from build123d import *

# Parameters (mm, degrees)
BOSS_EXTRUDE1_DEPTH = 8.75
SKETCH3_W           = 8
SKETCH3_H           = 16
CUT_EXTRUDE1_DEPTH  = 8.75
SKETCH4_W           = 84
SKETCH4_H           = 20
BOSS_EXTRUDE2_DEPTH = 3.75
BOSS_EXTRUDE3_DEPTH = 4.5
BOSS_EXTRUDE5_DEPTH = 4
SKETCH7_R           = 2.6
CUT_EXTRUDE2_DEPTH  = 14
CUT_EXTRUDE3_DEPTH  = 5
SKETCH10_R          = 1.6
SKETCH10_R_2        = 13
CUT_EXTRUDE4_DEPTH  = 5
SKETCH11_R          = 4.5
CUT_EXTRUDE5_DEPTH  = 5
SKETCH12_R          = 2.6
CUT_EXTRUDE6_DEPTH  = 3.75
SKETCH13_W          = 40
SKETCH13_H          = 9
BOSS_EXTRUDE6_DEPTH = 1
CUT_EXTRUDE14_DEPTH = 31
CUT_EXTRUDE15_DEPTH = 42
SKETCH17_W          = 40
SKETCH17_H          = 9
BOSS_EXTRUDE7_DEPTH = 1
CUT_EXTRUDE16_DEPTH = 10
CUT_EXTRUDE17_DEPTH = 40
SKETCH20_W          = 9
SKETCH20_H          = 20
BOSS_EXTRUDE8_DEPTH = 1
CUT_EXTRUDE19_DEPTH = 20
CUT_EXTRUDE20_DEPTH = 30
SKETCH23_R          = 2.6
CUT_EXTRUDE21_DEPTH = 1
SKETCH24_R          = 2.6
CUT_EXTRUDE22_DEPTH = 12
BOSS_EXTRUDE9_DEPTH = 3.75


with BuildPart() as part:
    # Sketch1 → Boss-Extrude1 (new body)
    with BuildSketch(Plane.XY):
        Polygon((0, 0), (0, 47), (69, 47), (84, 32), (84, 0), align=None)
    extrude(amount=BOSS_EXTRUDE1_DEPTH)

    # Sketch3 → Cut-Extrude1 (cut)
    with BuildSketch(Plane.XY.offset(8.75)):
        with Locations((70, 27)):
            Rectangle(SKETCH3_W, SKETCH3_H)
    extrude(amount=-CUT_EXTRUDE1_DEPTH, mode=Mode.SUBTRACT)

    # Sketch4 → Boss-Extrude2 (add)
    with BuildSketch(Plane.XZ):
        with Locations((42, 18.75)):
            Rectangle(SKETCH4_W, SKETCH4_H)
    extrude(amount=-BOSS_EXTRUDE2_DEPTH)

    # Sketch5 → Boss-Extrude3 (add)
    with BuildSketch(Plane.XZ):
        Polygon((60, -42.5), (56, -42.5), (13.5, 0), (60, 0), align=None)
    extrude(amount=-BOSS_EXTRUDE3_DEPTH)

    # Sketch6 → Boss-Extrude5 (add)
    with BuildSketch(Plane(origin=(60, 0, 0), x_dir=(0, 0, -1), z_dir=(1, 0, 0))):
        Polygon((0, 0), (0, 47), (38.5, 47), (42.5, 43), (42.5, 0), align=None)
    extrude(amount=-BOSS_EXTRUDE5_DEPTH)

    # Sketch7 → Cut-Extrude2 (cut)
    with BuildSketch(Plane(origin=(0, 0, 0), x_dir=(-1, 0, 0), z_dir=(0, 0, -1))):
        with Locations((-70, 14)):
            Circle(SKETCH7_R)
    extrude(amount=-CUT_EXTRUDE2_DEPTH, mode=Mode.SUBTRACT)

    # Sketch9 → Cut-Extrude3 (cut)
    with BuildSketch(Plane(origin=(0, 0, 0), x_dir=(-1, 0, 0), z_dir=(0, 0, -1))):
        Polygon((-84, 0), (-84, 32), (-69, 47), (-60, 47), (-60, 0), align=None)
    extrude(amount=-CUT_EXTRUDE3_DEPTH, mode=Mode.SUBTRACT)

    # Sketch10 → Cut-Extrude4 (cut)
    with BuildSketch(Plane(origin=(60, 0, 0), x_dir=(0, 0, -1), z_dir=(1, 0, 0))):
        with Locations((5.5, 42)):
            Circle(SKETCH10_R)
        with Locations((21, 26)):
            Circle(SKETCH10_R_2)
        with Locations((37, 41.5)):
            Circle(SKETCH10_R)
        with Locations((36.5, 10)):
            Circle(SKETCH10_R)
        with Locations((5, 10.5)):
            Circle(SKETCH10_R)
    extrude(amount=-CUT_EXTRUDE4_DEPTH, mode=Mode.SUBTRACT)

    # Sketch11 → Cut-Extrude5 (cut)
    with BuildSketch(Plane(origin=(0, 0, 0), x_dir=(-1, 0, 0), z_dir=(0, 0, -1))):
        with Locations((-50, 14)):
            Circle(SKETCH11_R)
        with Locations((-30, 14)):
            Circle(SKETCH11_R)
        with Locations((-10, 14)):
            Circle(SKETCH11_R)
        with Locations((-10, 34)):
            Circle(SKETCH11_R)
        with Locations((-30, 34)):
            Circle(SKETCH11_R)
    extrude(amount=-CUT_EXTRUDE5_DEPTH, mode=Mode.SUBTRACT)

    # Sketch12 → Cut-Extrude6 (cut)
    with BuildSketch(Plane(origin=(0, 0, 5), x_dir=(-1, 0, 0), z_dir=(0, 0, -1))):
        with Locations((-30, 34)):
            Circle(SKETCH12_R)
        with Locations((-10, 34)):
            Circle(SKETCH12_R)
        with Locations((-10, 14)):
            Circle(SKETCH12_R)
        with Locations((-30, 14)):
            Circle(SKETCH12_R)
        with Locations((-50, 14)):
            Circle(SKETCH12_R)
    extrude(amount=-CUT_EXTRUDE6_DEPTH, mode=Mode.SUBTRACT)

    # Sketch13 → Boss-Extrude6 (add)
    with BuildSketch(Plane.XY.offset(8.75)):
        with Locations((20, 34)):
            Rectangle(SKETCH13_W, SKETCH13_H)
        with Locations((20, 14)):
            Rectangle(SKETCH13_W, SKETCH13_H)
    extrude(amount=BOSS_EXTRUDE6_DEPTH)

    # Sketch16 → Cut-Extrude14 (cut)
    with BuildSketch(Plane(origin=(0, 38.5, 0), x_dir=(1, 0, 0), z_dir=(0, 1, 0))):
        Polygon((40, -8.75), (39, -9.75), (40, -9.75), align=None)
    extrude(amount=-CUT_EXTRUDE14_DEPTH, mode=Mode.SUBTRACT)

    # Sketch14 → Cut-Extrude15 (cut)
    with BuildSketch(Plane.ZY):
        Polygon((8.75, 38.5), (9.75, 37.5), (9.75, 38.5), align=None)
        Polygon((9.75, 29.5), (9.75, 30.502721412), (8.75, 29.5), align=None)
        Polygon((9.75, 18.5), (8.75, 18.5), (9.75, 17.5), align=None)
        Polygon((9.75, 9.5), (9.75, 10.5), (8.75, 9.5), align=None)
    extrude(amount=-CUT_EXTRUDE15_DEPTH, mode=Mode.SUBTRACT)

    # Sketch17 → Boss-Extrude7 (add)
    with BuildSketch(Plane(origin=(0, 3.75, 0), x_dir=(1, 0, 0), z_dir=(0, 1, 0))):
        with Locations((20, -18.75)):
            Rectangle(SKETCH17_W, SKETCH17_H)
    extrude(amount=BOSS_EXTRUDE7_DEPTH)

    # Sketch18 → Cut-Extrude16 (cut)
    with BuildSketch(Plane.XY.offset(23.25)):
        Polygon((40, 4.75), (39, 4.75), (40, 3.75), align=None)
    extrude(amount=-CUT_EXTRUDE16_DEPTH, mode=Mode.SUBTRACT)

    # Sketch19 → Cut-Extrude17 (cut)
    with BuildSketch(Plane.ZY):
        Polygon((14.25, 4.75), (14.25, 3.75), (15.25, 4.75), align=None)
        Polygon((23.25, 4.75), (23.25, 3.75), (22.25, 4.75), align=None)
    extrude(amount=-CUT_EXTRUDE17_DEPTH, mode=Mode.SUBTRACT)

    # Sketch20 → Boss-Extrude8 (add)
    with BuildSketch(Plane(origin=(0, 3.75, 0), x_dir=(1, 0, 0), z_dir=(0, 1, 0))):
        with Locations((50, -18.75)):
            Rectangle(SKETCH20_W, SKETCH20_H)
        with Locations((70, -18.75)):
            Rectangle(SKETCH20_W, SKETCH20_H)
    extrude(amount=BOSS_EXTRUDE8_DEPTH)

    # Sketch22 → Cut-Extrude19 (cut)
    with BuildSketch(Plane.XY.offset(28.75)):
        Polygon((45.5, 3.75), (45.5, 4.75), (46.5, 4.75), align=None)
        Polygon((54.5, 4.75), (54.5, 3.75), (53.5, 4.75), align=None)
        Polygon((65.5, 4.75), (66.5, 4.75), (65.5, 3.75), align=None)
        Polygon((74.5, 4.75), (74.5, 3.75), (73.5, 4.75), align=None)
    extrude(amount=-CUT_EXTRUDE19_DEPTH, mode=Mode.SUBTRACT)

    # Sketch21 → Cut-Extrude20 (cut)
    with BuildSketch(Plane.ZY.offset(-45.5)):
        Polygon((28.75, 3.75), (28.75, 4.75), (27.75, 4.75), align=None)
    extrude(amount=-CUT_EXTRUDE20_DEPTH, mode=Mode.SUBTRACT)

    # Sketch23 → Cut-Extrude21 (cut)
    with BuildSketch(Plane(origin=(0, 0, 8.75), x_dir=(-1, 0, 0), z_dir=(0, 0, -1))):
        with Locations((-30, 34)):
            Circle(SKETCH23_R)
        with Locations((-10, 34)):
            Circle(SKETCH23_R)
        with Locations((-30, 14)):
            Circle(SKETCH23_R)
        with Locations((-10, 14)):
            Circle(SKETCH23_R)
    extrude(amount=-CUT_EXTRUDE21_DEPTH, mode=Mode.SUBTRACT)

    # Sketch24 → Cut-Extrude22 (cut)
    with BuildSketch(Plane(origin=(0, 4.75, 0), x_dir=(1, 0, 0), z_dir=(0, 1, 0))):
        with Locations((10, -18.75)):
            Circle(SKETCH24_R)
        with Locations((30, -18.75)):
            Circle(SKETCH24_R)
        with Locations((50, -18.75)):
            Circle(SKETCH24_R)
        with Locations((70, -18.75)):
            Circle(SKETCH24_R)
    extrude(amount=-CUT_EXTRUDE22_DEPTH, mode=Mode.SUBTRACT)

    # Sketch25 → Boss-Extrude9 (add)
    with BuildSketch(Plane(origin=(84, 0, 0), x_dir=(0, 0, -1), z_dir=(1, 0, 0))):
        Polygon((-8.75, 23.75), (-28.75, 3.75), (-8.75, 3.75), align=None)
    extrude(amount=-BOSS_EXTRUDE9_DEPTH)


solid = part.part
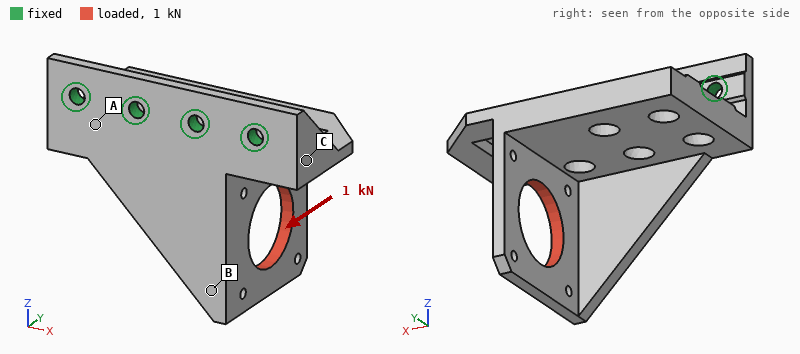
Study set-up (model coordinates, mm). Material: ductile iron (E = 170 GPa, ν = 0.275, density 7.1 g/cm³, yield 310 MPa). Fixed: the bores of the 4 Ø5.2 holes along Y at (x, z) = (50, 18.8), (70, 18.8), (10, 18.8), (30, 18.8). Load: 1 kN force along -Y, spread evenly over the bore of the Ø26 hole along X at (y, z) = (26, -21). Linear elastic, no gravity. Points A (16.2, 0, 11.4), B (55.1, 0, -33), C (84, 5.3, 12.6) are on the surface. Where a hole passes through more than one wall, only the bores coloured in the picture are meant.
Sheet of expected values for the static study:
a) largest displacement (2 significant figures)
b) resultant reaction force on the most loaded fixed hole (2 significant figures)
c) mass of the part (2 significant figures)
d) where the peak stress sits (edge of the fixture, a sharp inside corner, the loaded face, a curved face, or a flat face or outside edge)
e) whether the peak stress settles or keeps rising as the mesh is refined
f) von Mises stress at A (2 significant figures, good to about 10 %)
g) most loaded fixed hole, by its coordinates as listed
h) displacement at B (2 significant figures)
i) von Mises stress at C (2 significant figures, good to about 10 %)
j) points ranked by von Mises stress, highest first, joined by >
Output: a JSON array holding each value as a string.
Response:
["0.32 mm", "610 N", "310 g", "edge of the fixture", "keeps rising", "110 MPa", "(70, 18.8)", "0.21 mm", "39 MPa", "A > C > B"]
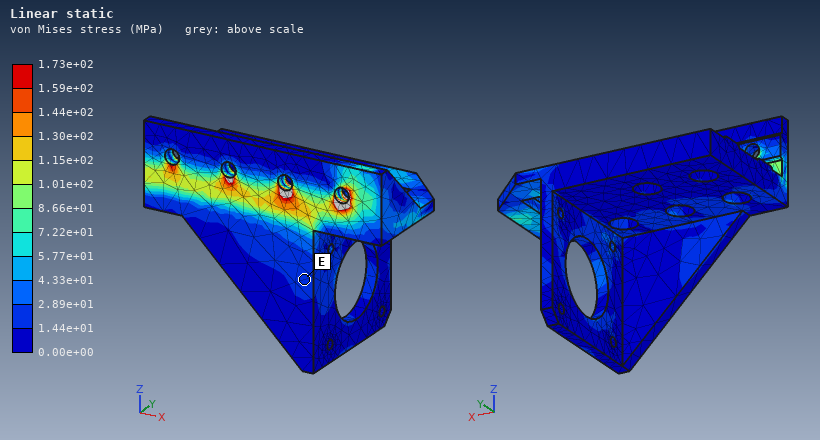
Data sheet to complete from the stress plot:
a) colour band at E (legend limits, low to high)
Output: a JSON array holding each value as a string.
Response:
["1.44e+01 to 2.89e+01 MPa"]
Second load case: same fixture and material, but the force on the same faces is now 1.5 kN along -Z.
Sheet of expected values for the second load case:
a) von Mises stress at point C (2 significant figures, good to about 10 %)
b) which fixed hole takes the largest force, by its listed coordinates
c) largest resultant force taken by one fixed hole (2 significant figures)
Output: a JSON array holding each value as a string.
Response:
["44 MPa", "(50, 18.8)", "860 N"]
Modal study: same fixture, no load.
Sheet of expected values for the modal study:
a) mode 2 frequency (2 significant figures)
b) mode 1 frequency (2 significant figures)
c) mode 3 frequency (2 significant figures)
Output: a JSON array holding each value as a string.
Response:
["2400 Hz", "910 Hz", "3100 Hz"]
